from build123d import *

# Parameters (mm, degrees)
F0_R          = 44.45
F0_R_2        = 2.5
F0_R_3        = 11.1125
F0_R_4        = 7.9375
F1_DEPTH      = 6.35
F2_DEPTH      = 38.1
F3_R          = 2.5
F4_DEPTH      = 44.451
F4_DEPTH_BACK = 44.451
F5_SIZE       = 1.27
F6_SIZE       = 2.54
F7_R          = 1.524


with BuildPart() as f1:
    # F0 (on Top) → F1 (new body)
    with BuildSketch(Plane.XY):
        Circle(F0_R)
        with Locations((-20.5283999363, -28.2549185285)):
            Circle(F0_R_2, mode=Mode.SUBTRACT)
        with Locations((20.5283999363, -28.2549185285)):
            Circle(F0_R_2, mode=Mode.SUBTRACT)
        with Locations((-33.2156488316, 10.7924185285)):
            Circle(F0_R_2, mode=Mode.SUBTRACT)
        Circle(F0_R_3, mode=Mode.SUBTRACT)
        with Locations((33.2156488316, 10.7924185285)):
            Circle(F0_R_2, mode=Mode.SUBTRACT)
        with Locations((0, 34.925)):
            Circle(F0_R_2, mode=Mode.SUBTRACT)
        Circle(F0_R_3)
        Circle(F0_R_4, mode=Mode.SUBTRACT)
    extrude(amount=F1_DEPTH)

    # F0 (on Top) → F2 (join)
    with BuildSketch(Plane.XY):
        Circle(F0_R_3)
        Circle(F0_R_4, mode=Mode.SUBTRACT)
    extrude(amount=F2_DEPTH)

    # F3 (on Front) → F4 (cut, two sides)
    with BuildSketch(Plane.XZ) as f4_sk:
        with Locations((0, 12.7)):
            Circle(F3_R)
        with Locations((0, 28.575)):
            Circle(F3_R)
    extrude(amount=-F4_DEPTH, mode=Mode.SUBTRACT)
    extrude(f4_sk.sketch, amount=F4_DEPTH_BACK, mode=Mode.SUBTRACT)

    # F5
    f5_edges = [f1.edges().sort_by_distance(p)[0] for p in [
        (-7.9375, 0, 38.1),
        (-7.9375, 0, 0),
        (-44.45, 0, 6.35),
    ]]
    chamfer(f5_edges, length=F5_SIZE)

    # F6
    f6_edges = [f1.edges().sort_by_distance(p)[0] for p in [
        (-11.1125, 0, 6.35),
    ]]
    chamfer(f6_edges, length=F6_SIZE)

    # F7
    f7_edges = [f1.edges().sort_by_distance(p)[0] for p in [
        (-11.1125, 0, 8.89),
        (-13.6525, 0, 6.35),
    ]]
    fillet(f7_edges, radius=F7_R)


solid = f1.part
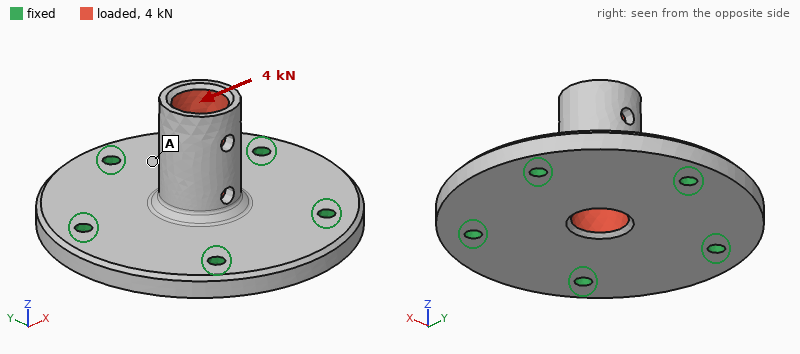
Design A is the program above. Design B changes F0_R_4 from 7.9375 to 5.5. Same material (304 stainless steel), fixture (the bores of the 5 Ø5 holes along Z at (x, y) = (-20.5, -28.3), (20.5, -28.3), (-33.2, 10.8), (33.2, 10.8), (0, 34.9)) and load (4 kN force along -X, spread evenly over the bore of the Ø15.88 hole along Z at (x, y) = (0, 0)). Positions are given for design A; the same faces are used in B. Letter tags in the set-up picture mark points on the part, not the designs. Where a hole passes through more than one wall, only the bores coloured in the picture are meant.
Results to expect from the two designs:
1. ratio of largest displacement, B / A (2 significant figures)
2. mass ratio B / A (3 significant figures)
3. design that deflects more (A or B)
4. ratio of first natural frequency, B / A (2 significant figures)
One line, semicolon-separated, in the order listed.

0.81; 1.09; A; 0.91
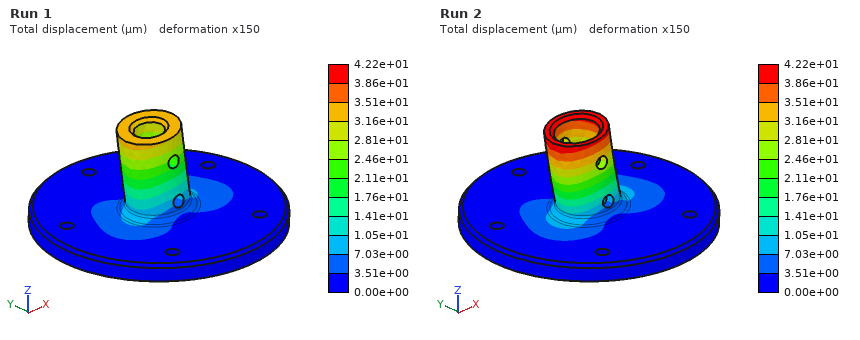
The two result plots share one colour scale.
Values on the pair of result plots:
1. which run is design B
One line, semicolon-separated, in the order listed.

Run 1
